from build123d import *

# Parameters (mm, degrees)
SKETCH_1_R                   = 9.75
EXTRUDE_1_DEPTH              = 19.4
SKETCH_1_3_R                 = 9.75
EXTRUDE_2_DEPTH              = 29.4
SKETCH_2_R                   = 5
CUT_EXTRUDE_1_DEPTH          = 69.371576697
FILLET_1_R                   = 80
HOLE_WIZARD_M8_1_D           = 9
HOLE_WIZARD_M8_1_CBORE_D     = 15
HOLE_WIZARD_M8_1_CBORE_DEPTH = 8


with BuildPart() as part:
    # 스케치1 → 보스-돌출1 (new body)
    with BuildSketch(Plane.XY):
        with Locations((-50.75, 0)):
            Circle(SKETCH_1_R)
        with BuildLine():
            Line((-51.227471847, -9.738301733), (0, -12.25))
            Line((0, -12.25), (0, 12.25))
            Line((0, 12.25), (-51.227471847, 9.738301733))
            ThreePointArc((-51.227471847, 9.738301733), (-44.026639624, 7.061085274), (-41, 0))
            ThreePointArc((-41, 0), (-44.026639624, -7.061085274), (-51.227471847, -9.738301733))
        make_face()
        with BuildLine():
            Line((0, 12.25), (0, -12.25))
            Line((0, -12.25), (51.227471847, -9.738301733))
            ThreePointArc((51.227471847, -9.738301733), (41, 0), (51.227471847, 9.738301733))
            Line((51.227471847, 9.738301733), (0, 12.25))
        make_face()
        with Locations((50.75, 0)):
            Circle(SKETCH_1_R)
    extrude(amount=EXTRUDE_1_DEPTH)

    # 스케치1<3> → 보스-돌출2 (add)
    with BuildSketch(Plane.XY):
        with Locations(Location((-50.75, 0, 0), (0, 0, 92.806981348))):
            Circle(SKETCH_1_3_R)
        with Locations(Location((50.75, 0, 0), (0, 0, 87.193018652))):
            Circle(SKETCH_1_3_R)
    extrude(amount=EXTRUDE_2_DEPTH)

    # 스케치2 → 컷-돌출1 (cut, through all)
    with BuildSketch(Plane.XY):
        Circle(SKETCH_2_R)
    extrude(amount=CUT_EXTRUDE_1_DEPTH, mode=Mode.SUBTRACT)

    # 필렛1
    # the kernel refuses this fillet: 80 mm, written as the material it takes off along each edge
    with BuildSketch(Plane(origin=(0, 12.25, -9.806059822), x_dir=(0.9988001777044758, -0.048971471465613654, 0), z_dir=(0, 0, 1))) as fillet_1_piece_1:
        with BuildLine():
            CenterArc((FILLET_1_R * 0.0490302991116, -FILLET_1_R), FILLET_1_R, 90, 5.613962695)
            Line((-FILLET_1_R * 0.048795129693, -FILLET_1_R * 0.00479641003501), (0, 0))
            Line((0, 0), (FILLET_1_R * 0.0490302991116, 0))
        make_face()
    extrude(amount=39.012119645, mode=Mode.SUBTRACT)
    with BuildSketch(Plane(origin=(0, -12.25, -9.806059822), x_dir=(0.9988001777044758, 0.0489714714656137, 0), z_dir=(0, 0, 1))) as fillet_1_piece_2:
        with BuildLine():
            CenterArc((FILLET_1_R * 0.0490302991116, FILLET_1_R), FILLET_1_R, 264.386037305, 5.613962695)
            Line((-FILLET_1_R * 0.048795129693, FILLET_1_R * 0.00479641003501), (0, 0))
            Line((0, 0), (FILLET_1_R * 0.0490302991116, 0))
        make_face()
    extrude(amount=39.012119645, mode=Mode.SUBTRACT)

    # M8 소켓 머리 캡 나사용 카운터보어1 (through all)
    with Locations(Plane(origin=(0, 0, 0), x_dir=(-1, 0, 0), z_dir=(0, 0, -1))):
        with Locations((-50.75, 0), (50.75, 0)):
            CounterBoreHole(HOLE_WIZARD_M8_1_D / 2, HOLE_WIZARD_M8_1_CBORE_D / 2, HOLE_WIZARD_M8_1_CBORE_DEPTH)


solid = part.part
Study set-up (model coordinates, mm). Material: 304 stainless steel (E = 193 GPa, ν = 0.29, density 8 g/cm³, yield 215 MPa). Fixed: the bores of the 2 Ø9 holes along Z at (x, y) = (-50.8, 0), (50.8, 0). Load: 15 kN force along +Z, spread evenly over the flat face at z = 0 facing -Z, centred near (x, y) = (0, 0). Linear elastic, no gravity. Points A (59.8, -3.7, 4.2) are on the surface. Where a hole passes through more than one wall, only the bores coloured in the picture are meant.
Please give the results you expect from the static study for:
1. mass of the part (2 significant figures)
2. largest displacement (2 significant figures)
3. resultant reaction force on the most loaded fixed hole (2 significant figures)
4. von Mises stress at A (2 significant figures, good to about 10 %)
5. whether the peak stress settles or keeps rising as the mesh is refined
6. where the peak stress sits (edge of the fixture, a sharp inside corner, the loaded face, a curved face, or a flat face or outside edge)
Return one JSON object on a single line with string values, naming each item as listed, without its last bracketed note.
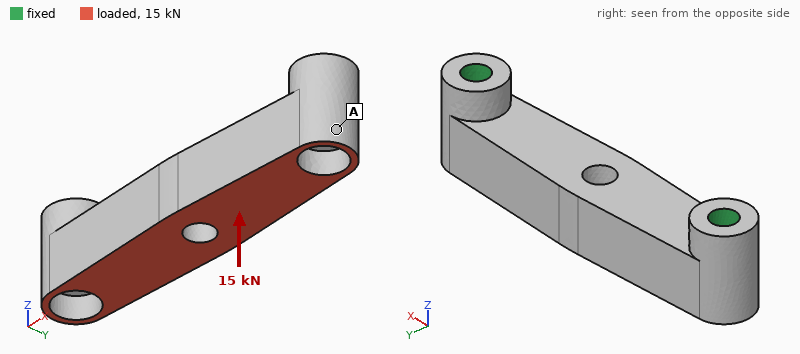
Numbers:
{"mass of the part": "380 g", "largest displacement": "30 µm", "resultant reaction force on the most loaded fixed hole": "8.5 kN", "von Mises stress at A": "24 MPa", "whether the peak stress settles or keeps rising as the mesh is refined": "keeps rising", "where the peak stress sits": "edge of the fixture"}
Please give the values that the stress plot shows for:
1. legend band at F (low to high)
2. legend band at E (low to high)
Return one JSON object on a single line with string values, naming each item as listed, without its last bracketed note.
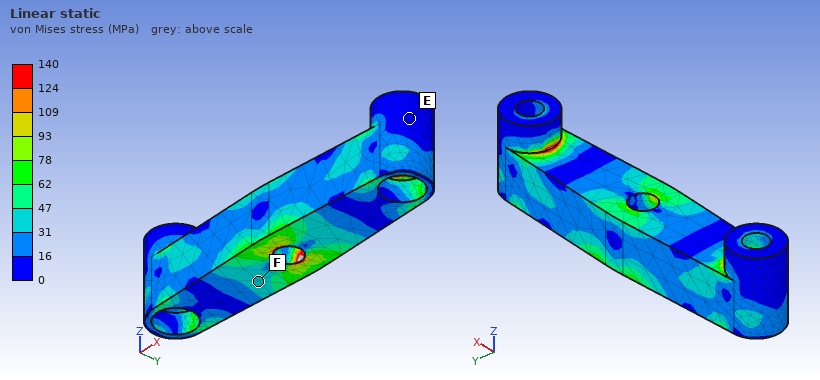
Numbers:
{"legend band at F": "31 to 47 MPa", "legend band at E": "0 to 16 MPa"}
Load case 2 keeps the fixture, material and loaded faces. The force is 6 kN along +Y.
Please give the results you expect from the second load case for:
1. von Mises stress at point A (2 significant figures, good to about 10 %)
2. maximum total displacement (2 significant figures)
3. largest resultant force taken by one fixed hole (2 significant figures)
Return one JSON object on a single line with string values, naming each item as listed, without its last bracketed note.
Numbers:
{"von Mises stress at point A": "10 MPa", "maximum total displacement": "19 µm", "largest resultant force taken by one fixed hole": "3.0 kN"}
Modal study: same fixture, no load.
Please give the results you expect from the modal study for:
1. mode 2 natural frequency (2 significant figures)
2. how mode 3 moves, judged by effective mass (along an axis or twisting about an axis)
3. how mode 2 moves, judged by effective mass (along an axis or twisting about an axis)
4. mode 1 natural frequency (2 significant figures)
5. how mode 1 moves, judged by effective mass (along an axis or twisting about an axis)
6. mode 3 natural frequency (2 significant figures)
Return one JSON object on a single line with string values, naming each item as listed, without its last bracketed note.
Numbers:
{"mode 2 natural frequency": "7500 Hz", "how mode 3 moves, judged by effective mass": "twisting about X", "how mode 2 moves, judged by effective mass": "along Y", "mode 1 natural frequency": "7100 Hz", "how mode 1 moves, judged by effective mass": "along Z", "mode 3 natural frequency": "12 kHz"}
